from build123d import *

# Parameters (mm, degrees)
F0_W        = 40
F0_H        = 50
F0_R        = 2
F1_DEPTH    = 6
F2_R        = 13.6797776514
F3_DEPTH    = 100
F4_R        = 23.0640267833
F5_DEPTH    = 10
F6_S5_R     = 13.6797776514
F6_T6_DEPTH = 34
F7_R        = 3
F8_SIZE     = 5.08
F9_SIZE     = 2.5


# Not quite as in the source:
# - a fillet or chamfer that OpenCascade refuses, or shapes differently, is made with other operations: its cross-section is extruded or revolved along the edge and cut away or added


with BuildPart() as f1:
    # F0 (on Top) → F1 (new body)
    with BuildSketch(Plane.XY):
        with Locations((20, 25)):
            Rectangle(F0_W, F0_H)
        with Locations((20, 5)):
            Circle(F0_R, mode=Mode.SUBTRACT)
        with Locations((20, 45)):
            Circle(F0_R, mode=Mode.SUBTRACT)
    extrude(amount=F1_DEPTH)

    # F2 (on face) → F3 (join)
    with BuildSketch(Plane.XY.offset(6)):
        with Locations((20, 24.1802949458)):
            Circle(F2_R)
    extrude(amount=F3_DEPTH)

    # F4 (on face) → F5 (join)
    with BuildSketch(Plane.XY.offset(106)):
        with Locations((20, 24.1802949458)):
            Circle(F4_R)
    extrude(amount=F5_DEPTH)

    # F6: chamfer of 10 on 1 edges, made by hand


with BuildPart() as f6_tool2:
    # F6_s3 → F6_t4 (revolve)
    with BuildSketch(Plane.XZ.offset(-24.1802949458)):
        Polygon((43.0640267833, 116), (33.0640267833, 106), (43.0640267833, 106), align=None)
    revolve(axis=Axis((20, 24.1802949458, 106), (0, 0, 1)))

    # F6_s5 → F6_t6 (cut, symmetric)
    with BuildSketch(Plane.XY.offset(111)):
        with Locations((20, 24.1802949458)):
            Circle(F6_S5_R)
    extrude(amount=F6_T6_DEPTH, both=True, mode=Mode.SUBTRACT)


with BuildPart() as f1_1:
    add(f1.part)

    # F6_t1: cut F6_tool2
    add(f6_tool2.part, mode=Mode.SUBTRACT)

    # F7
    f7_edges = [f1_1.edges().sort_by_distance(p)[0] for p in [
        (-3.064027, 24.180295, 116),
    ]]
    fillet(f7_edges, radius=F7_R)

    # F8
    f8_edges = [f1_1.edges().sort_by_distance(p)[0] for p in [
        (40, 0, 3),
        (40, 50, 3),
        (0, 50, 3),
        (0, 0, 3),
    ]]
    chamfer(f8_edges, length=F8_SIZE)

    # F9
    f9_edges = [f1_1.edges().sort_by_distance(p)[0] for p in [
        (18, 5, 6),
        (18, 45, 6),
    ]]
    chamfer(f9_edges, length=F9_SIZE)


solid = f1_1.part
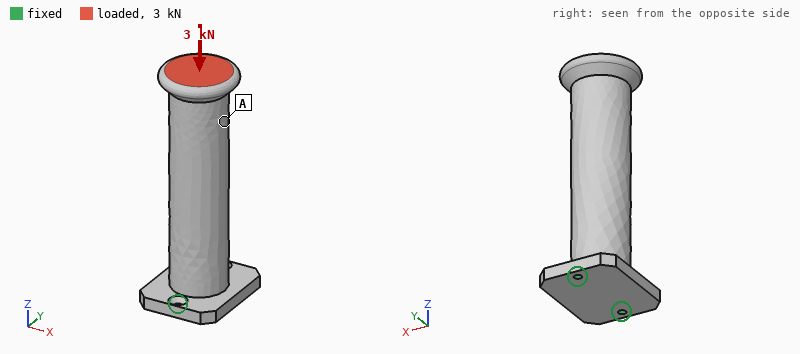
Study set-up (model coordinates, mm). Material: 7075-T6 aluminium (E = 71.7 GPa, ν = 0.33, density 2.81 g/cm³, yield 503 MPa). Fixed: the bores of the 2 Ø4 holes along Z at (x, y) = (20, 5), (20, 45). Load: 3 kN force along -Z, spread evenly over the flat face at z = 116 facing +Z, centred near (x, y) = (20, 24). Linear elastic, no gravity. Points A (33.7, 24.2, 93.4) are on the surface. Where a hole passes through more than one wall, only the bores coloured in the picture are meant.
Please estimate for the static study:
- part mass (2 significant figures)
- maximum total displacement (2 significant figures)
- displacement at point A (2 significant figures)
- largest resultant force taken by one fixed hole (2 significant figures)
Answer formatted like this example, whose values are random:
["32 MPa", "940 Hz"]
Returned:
["220 g", "25 µm", "22 µm", "1.8 kN"]
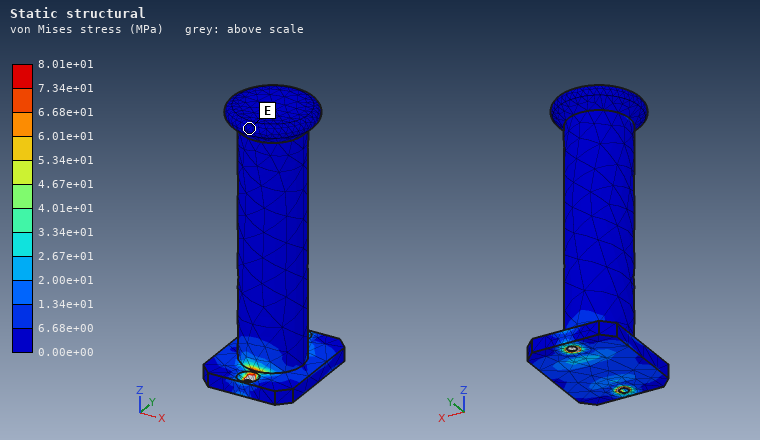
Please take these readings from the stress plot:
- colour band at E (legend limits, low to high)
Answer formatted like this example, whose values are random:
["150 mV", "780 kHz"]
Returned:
["0.00e+00 to 6.68e+00 MPa"]
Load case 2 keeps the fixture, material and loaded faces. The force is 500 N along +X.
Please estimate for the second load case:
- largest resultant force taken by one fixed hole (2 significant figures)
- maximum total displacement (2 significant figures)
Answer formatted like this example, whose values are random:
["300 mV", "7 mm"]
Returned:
["260 N", "1.4 mm"]
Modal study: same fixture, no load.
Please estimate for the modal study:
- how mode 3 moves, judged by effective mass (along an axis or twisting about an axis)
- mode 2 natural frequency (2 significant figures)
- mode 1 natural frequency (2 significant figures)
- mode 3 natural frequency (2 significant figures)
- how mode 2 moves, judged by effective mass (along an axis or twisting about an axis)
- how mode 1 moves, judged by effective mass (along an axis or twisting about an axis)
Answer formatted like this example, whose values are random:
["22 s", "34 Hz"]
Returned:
["along Z", "1000 Hz", "360 Hz", "4700 Hz", "along Y", "along X"]
